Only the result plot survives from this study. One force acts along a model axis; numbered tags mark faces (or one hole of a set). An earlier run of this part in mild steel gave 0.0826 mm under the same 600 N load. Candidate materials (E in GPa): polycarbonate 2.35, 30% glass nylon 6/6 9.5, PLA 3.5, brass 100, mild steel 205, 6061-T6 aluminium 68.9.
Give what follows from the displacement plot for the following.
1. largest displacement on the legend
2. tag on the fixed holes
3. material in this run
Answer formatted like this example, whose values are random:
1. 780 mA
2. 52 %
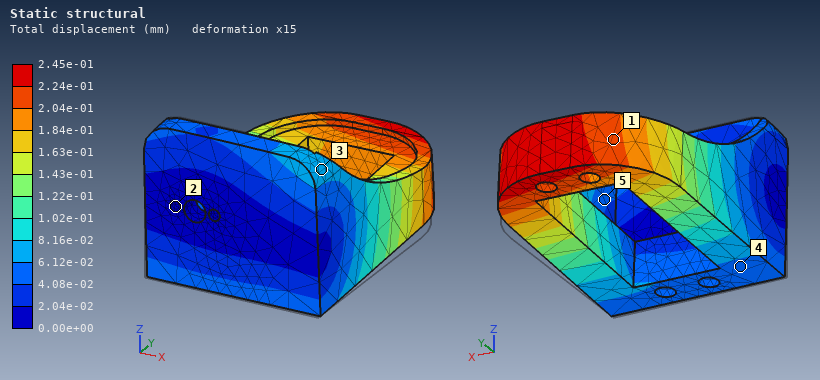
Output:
1. 2.45e-01 mm
2. 2
3. 6061-T6 aluminium
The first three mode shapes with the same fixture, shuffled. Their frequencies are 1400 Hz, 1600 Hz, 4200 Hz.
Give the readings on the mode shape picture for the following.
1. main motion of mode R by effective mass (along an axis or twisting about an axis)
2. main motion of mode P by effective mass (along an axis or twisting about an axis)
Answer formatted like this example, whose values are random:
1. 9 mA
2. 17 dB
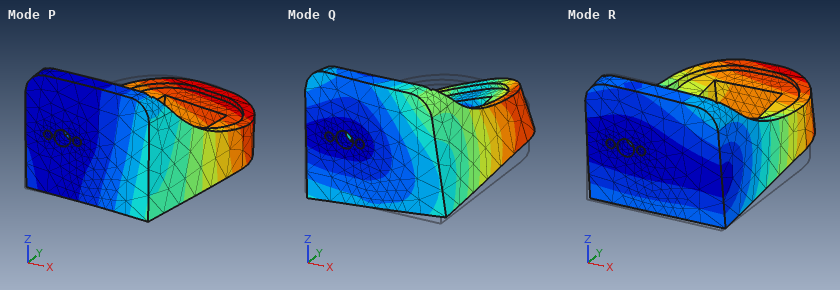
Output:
1. along Z
2. along X
